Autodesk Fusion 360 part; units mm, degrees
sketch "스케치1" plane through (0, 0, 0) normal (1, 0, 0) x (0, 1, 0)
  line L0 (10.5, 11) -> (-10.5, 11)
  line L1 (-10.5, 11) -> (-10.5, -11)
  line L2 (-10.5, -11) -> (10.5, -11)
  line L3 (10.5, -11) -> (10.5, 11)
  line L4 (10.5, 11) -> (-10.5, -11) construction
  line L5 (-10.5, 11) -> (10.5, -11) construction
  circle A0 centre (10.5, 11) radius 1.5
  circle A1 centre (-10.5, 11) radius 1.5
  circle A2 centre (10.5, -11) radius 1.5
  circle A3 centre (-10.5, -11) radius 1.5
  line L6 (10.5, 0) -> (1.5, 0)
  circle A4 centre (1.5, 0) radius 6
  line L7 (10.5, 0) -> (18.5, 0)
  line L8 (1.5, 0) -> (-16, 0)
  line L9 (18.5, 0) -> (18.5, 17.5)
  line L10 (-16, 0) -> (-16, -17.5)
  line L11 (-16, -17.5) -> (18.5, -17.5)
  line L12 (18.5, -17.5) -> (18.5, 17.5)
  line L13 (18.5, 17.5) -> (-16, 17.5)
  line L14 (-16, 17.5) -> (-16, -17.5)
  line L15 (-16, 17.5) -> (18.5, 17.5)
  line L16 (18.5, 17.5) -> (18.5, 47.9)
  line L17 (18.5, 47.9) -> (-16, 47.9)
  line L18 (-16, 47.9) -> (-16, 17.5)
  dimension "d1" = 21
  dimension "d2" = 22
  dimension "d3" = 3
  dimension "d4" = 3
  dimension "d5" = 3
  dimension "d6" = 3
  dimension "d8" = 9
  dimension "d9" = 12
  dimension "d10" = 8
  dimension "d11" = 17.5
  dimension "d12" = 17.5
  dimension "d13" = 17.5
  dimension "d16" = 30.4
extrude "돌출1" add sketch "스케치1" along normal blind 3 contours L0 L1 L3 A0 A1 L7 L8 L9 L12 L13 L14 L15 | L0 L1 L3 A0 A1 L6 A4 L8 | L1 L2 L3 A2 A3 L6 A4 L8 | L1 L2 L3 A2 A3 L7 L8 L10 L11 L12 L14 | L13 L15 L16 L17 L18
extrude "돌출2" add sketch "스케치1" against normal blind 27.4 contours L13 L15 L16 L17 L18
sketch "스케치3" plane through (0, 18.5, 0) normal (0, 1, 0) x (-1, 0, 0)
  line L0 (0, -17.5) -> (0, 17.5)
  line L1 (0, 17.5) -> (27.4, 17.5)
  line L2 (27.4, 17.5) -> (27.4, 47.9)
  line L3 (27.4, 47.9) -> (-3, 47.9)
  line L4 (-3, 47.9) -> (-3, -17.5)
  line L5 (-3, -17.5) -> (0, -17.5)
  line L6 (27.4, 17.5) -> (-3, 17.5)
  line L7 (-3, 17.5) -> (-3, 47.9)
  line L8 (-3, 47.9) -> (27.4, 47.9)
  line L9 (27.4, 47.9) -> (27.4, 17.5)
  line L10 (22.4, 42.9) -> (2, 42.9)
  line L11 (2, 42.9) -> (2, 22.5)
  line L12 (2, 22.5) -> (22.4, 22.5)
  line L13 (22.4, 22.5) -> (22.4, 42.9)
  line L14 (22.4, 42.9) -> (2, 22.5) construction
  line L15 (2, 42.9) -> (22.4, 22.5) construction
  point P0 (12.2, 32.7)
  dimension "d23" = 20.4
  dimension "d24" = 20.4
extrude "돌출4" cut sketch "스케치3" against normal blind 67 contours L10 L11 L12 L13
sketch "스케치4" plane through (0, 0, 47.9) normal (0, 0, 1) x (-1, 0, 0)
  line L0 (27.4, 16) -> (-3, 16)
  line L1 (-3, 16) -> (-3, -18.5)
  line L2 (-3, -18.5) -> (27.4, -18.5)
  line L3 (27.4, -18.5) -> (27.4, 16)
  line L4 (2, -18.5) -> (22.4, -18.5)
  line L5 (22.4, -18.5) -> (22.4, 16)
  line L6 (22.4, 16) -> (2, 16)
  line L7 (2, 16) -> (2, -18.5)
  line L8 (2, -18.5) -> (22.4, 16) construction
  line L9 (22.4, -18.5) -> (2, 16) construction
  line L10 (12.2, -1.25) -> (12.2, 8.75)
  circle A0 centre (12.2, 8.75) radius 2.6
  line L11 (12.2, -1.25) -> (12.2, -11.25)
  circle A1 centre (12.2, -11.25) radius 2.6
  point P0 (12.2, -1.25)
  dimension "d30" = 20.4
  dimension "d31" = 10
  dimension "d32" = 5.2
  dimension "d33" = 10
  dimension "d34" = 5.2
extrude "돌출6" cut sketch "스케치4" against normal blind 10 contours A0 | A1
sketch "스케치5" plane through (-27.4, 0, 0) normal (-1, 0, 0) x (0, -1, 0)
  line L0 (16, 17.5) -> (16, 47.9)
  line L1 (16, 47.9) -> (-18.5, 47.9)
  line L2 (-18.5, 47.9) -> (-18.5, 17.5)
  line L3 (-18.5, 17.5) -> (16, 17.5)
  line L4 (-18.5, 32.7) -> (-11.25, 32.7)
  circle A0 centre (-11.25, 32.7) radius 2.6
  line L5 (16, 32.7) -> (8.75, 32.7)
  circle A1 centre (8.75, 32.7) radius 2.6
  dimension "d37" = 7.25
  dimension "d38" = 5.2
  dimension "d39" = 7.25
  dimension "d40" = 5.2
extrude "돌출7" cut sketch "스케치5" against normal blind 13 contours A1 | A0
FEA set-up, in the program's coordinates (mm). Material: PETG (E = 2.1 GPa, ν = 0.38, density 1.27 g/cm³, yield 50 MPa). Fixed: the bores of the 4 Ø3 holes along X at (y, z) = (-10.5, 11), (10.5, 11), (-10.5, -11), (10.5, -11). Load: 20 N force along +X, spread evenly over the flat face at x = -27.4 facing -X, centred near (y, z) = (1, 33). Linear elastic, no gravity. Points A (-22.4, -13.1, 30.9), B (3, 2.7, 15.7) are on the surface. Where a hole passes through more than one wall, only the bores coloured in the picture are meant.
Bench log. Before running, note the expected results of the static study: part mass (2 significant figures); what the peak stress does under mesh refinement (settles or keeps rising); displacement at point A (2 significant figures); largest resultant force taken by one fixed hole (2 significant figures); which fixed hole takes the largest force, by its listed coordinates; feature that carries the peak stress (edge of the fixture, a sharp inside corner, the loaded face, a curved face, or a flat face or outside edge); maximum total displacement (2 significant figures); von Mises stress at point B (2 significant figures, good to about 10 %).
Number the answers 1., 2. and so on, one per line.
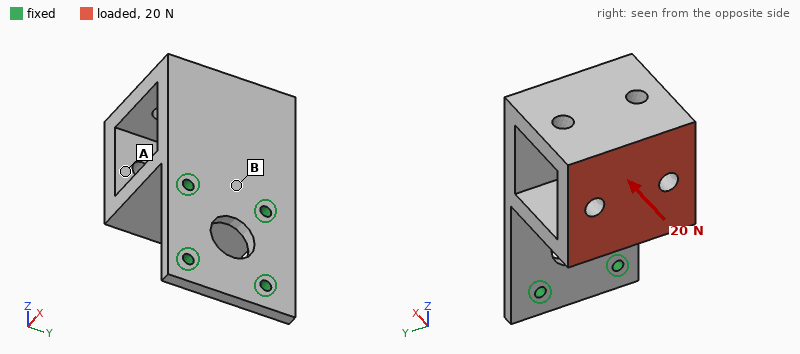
1. 26 g
2. keeps rising
3. 0.51 mm
4. 13 N
5. (10.5, 11)
6. edge of the fixture
7. 0.78 mm
8. 5.0 MPa
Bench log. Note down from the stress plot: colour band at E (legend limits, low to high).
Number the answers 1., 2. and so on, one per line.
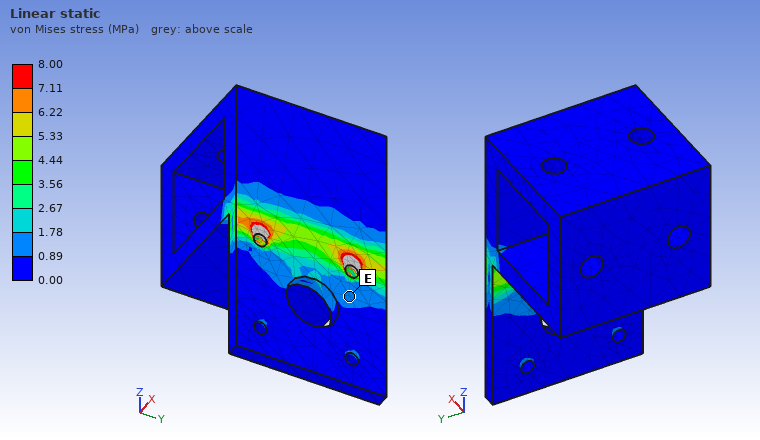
1. 0.89 to 1.78 MPa
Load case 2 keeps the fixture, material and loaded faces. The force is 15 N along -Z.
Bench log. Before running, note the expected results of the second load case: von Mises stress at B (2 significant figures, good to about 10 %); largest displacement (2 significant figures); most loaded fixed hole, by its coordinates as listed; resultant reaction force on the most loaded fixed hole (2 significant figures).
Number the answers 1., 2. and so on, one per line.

1. 6.5 MPa
2. 0.95 mm
3. (10.5, 11)
4. 7.8 N
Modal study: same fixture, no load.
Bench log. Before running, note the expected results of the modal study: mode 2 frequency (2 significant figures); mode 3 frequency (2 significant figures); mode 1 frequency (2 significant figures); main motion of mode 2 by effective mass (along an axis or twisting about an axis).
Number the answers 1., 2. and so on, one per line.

1. 760 Hz
2. 1500 Hz
3. 180 Hz
4. along Y
